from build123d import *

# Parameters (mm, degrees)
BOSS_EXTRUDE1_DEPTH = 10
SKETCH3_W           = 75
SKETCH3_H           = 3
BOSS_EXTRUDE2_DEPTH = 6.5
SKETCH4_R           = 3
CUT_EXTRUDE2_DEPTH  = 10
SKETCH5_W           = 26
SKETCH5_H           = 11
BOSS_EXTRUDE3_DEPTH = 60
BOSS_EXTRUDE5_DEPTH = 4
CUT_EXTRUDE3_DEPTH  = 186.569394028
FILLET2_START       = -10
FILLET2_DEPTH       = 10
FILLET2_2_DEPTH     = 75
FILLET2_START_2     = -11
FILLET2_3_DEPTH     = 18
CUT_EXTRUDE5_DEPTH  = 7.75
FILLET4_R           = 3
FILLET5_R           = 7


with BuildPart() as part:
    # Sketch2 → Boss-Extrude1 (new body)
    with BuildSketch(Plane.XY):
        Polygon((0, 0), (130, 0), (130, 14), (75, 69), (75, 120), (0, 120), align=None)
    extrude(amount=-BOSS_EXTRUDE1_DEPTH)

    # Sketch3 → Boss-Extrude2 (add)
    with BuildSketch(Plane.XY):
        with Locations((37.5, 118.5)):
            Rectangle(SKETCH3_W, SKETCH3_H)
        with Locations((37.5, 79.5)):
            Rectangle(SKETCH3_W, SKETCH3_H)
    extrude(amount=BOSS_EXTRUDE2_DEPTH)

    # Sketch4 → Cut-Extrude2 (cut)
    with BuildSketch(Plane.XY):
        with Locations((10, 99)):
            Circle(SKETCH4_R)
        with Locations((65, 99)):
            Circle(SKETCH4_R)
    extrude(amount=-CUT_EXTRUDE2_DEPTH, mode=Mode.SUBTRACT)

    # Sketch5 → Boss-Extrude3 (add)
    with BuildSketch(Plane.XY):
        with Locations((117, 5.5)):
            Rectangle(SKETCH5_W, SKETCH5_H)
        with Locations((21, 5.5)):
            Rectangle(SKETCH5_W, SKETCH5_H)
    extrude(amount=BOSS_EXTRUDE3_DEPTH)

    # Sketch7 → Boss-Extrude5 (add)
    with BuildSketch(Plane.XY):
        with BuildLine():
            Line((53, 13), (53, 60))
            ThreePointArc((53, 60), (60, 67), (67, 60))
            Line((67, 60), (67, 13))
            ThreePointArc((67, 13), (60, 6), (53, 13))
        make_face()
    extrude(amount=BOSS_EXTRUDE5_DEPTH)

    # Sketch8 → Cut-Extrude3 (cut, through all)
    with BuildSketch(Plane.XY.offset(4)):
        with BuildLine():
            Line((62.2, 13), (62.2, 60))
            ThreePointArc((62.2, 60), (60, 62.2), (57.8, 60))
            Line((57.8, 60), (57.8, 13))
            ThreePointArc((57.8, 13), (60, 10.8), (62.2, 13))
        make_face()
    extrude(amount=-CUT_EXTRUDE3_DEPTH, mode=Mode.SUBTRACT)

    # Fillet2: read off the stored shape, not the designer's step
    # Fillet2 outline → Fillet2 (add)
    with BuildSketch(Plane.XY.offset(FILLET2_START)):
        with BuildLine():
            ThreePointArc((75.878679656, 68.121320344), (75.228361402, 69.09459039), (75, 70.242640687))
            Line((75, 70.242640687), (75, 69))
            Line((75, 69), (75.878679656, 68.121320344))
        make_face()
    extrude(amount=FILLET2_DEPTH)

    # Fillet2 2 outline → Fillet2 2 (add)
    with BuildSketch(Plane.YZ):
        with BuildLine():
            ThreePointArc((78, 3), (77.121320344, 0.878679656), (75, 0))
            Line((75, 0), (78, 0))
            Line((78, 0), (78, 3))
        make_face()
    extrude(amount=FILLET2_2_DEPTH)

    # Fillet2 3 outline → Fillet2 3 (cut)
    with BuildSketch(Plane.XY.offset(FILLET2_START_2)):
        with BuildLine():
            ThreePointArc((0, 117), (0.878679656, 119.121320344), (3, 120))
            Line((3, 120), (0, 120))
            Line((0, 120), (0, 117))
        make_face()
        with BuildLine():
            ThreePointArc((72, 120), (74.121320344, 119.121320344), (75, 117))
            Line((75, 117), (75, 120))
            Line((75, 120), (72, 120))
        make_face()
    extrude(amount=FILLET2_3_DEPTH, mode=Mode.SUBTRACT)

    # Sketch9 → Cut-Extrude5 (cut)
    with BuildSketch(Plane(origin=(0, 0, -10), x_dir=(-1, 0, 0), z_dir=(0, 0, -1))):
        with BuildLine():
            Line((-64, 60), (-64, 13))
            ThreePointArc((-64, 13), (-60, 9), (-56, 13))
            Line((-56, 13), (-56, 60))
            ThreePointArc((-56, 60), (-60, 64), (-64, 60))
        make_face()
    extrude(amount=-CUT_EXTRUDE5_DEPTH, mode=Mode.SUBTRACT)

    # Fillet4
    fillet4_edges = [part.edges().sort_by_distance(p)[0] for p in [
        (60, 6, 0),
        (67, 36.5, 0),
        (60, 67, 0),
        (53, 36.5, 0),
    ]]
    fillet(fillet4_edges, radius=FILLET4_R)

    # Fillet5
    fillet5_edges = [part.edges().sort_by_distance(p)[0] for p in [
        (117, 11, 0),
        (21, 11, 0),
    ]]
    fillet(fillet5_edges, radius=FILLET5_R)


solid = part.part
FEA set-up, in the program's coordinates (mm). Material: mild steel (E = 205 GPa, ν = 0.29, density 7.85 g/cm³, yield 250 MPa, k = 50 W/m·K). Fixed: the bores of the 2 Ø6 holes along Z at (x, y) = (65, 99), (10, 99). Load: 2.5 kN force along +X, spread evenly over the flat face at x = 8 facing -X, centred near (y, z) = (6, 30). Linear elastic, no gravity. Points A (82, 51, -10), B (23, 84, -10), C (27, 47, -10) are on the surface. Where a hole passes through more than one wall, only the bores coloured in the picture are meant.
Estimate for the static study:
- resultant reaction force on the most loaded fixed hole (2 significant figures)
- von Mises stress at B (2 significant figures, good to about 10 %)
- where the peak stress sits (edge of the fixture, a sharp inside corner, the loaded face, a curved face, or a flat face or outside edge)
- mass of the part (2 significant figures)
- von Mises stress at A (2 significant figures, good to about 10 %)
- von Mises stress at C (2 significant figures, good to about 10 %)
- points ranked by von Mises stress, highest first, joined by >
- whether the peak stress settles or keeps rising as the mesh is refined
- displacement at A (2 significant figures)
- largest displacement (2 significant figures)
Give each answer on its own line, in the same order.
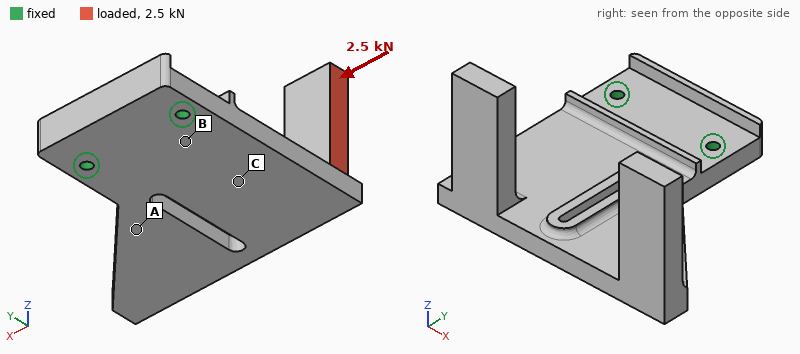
4.6 kN
39 MPa
edge of the fixture
1.2 kg
17 MPa
60 MPa
C > B > A
keeps rising
0.057 mm
0.32 mm
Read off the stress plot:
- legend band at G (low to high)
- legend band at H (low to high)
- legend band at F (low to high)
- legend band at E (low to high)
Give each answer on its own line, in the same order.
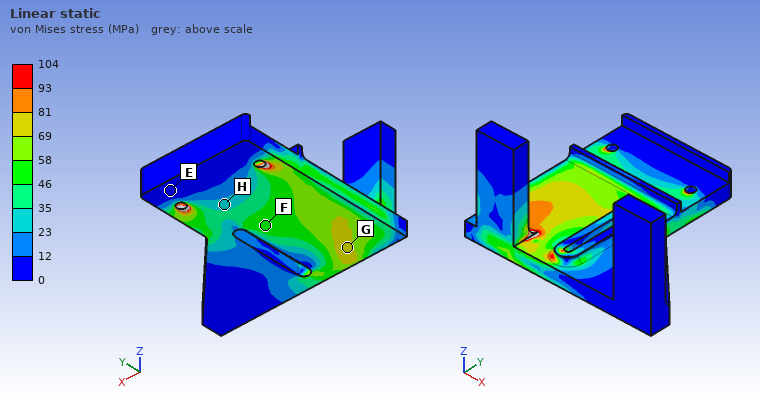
69 to 81 MPa
23 to 35 MPa
46 to 58 MPa
0 to 12 MPa
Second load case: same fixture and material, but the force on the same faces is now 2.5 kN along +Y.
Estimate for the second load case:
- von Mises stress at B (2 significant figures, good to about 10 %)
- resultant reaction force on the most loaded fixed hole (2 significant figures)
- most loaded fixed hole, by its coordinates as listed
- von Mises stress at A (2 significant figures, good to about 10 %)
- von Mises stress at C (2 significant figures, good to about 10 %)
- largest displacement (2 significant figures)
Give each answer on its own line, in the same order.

55 MPa
2.6 kN
(10, 99)
32 MPa
56 MPa
0.66 mm
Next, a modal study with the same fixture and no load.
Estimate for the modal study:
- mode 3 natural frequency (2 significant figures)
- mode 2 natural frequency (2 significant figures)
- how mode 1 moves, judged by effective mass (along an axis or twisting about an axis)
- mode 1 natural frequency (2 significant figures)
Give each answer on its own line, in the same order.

1200 Hz
650 Hz
along Z
380 Hz
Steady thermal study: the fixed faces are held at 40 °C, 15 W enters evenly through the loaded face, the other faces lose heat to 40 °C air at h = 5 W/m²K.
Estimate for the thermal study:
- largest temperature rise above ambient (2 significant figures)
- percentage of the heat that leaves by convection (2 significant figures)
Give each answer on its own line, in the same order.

70 K
23 %
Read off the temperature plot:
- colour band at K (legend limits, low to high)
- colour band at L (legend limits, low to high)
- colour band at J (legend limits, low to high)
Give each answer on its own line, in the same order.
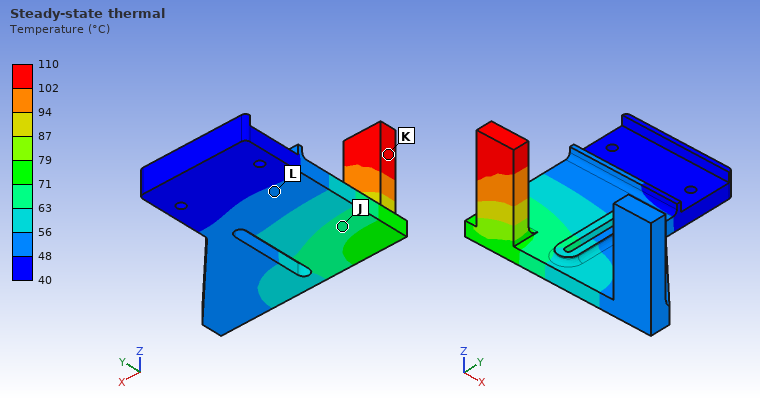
102 to 110 °C
48 to 56 °C
63 to 71 °C
